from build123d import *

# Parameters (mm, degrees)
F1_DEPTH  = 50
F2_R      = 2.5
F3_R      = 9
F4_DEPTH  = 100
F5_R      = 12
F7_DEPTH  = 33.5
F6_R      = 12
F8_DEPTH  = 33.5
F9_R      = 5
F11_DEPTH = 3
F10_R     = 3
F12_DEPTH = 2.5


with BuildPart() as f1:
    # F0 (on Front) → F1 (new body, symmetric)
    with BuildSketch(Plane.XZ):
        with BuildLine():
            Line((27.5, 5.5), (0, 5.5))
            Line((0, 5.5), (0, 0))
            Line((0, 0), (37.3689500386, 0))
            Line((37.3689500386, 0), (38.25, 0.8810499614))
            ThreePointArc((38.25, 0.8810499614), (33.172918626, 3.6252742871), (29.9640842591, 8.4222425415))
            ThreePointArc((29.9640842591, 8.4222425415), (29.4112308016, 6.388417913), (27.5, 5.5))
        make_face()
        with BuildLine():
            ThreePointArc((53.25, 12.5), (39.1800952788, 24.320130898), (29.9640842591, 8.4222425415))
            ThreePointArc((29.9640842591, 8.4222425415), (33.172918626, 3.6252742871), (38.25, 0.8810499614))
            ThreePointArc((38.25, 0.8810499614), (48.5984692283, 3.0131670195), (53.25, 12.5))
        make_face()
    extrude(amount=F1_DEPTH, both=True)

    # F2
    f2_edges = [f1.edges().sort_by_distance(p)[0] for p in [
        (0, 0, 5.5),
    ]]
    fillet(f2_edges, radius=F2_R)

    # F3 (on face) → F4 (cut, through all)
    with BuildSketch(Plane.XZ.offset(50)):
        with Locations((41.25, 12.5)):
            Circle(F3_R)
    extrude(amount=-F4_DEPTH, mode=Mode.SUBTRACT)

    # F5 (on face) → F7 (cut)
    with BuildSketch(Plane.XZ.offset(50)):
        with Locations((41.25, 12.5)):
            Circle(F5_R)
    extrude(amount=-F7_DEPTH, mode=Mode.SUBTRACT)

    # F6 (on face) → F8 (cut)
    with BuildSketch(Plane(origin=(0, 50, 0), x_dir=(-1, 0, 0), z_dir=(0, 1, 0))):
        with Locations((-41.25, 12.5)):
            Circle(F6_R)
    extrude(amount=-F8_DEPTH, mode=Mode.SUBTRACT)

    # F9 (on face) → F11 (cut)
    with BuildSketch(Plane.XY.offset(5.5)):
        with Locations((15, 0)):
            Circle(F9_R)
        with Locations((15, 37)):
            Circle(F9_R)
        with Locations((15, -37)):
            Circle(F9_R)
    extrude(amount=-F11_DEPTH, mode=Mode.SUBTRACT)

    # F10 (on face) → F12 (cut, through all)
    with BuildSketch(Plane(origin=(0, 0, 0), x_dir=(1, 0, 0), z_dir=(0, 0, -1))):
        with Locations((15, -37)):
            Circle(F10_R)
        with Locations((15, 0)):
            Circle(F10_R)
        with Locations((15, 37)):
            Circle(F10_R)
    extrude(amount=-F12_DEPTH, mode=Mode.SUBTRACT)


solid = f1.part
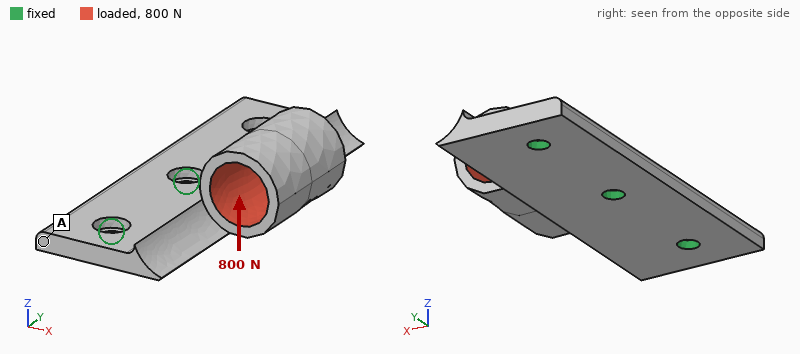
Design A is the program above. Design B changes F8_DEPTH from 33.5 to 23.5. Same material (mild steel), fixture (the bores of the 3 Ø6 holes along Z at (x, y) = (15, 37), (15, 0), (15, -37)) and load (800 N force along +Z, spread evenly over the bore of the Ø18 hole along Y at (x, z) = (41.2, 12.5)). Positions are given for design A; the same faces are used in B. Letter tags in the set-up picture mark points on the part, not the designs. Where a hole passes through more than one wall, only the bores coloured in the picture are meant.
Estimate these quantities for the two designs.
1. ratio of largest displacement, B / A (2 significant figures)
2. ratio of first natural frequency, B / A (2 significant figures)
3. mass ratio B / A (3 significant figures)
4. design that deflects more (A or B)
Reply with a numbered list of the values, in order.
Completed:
1. 0.89
2. 0.94
3. 1.08
4. A
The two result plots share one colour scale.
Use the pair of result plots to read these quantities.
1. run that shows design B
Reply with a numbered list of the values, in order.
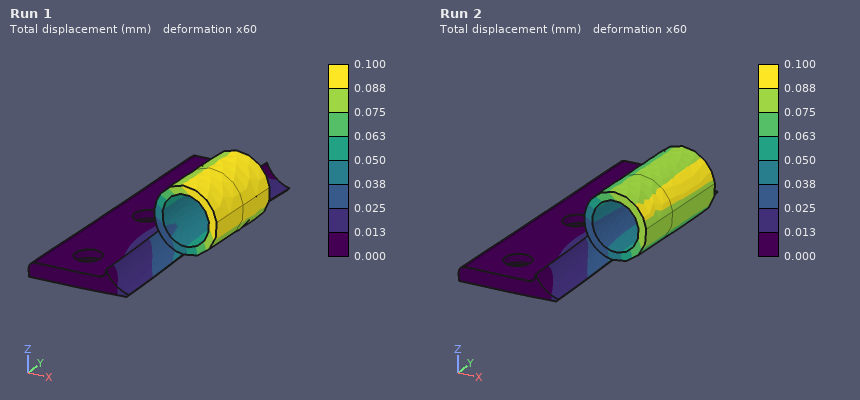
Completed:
1. Run 2
